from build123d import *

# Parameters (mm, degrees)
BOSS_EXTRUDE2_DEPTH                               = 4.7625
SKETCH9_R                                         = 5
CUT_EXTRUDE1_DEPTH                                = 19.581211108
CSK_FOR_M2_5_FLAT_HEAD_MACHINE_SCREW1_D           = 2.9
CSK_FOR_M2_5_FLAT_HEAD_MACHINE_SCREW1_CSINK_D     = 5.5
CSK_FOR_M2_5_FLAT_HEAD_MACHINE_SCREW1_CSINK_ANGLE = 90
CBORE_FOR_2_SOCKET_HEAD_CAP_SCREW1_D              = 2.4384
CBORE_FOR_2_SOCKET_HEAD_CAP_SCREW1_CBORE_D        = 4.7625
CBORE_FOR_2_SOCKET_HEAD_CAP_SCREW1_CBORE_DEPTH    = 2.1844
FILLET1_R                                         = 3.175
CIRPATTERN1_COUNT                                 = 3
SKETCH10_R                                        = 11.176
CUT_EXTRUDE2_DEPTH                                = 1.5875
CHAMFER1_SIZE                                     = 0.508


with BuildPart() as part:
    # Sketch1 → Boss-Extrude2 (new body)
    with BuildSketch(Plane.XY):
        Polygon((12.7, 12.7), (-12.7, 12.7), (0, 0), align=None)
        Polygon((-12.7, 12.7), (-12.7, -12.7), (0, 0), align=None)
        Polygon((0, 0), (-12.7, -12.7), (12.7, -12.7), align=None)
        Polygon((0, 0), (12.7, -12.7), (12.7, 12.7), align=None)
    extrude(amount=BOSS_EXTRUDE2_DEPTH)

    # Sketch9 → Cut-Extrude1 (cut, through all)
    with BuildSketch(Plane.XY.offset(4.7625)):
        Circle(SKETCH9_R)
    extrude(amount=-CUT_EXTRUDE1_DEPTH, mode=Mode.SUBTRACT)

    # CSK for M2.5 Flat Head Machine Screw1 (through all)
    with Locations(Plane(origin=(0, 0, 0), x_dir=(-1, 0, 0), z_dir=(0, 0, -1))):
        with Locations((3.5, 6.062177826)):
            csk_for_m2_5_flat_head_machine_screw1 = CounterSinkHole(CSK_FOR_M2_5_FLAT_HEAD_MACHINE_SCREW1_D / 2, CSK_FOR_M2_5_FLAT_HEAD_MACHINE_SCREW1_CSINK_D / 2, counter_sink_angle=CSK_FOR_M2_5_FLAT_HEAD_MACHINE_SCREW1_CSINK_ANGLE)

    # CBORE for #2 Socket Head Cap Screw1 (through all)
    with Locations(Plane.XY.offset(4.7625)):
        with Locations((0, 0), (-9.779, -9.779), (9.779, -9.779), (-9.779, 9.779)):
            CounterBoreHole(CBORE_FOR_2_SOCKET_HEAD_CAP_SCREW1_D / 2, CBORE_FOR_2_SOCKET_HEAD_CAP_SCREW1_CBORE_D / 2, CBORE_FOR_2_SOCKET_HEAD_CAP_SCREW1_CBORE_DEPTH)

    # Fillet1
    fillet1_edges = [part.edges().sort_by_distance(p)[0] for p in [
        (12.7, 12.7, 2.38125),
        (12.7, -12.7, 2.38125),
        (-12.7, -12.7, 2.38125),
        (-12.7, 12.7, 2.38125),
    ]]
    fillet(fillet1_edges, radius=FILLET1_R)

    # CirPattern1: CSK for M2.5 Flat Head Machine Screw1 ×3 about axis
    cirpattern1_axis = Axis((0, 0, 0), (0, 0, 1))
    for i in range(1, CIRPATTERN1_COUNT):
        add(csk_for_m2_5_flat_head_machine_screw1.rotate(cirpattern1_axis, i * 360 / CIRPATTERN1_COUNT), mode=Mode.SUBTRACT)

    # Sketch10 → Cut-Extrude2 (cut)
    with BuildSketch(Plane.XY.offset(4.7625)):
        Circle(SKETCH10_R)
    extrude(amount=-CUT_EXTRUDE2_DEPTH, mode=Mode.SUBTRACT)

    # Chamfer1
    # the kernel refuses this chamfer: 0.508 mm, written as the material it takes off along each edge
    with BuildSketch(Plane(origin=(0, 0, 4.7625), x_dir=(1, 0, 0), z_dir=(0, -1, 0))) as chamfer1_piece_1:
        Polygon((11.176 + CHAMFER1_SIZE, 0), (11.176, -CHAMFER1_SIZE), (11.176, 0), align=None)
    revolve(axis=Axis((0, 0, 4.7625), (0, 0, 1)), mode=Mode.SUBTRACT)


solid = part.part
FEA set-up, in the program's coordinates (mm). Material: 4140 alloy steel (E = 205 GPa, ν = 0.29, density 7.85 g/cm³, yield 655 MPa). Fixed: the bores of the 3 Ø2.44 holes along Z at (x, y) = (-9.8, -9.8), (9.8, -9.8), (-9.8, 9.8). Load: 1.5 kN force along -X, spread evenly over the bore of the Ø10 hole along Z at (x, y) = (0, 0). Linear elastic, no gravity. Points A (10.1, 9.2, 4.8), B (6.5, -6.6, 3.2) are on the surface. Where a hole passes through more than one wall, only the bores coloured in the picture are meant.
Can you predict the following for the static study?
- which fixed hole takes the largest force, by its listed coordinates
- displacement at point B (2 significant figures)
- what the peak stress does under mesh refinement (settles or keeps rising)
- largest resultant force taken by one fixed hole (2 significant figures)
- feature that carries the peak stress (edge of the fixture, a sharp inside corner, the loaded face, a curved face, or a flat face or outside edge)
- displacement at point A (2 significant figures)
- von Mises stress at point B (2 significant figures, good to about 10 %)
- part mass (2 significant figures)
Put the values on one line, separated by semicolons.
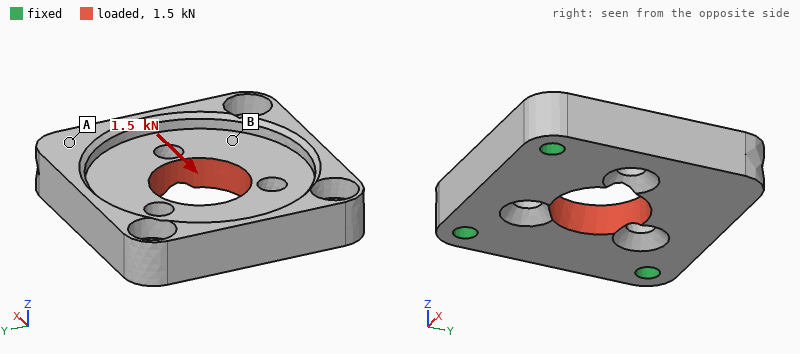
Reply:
(-9.8, 9.8); 0.92 µm; keeps rising; 670 N; a sharp inside corner; 1.6 µm; 19 MPa; 15 g
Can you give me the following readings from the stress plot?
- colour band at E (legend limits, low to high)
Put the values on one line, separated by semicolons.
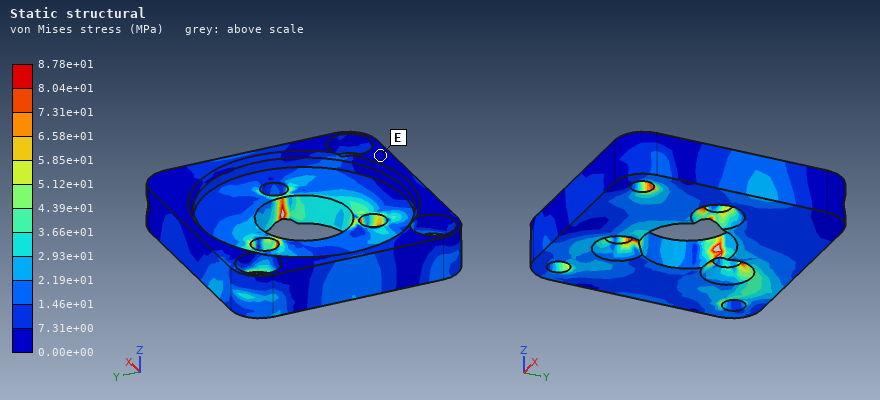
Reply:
0.00e+00 to 7.31e+00 MPa
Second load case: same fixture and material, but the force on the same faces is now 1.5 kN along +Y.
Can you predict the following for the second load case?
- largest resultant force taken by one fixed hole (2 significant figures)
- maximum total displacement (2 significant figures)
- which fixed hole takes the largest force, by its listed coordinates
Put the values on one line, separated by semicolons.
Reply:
660 N; 3.1 µm; (9.8, -9.8)
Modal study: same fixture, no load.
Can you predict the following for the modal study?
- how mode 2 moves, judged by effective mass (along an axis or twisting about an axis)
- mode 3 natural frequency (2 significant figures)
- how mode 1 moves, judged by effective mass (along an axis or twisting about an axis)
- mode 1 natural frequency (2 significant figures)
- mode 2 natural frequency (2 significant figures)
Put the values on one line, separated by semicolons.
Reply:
along Z; 30 kHz; along Z; 8300 Hz; 29 kHz
